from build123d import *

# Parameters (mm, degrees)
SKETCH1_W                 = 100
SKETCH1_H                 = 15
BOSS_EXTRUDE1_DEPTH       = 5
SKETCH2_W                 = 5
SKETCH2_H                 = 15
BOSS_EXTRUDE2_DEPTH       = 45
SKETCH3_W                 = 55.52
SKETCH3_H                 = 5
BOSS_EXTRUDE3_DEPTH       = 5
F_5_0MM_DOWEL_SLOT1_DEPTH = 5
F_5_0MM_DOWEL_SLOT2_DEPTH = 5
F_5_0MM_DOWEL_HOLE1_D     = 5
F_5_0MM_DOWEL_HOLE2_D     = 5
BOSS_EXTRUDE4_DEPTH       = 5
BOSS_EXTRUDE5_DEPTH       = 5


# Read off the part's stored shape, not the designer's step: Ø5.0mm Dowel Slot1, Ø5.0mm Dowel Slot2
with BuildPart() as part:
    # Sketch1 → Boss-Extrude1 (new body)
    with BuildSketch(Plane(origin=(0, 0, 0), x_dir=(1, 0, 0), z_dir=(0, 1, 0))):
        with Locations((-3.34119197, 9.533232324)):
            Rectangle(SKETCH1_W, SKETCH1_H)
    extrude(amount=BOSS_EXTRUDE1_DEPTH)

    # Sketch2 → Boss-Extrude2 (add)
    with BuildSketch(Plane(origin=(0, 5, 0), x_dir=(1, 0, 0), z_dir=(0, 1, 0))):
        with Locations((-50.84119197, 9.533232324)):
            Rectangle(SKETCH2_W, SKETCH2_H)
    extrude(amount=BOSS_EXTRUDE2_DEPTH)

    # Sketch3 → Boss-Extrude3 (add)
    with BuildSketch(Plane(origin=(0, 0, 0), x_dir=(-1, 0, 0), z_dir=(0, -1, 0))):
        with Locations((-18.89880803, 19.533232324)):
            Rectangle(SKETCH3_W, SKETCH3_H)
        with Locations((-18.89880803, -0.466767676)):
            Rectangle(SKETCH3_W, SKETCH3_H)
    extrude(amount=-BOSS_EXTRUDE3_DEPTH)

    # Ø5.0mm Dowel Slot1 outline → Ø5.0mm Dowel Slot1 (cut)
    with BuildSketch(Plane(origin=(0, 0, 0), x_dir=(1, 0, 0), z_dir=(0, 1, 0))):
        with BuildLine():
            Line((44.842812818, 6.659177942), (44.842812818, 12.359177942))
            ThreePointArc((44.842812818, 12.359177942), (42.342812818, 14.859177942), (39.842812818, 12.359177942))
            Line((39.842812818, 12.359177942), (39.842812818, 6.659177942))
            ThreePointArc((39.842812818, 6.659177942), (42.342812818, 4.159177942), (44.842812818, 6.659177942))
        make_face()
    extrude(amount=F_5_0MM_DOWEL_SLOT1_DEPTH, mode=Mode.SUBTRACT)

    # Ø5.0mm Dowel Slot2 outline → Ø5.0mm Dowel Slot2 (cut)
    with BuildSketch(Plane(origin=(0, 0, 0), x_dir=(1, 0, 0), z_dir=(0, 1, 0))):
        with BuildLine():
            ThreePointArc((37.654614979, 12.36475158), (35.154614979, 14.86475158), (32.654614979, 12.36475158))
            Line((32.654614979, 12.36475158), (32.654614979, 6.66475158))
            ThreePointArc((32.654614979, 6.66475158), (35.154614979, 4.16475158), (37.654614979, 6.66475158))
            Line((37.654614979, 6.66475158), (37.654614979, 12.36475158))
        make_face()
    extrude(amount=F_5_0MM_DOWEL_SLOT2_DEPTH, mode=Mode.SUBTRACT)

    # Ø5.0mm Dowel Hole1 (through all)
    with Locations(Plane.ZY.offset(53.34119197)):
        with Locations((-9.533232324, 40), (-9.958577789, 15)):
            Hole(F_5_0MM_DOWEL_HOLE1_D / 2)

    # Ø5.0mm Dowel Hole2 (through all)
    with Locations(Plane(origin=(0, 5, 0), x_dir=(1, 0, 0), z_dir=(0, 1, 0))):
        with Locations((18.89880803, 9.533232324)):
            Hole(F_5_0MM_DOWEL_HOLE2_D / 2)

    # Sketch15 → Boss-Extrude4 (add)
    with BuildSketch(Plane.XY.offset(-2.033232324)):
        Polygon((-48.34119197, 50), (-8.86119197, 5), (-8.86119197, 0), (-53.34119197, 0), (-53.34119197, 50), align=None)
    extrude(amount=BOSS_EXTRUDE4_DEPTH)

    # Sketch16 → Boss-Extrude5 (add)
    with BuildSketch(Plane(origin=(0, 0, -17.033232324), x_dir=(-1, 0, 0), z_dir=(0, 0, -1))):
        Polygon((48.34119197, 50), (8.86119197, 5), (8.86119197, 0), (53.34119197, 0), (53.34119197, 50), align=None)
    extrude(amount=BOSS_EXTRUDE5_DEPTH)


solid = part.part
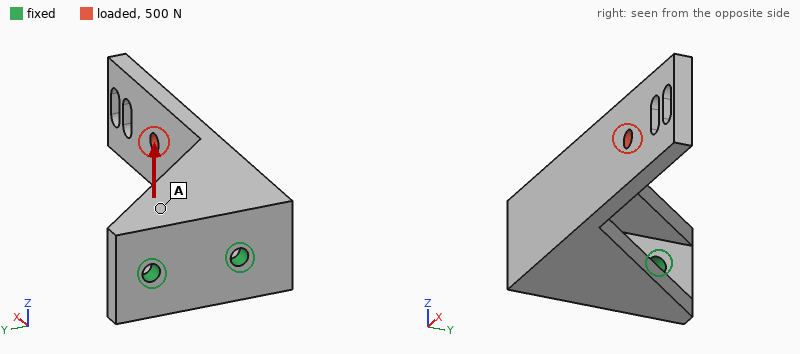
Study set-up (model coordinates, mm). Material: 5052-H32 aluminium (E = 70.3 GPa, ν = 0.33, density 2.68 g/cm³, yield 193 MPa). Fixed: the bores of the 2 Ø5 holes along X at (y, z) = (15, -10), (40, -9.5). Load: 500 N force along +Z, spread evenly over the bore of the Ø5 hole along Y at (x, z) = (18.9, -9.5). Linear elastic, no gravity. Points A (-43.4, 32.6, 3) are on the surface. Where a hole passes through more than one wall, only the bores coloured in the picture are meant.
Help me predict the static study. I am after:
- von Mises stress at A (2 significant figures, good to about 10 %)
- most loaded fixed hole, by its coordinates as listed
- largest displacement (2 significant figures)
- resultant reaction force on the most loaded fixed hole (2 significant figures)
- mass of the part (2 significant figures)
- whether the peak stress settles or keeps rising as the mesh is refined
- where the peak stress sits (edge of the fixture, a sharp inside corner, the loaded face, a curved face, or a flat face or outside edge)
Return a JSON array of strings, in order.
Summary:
["33 MPa", "(15, -10)", "0.56 mm", "660 N", "70 g", "keeps rising", "edge of the fixture"]
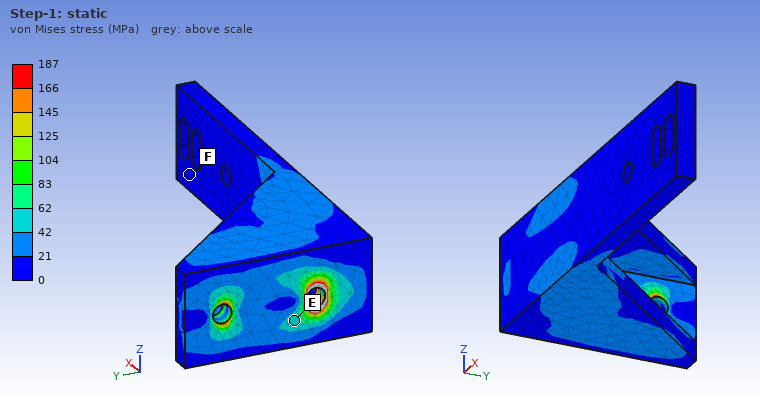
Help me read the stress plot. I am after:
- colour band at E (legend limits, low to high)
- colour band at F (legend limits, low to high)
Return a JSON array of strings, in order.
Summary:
["42 to 62 MPa", "0 to 21 MPa"]
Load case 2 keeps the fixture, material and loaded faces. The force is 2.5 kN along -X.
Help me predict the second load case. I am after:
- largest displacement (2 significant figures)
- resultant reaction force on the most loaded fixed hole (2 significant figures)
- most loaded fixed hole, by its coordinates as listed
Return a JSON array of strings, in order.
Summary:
["0.16 mm", "3.4 kN", "(15, -10)"]
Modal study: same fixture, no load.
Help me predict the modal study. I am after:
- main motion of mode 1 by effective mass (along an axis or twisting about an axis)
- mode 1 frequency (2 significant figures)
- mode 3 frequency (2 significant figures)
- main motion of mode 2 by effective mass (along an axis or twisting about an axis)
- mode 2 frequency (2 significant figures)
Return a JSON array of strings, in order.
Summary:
["along Y", "1100 Hz", "4600 Hz", "along Z", "1300 Hz"]
